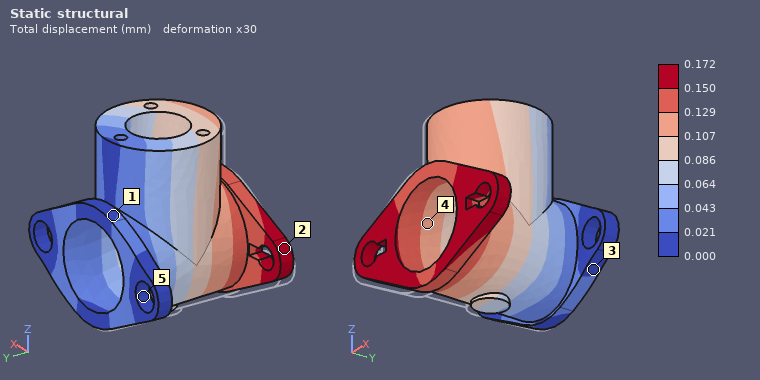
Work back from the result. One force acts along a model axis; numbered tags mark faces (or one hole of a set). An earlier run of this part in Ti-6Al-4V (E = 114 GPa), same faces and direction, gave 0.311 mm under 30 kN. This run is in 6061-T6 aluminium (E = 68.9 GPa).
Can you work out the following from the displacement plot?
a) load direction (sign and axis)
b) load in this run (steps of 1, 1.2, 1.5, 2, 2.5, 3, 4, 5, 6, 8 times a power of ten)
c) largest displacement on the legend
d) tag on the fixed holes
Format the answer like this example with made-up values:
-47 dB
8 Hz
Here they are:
+X
10 kN
0.172 mm
5
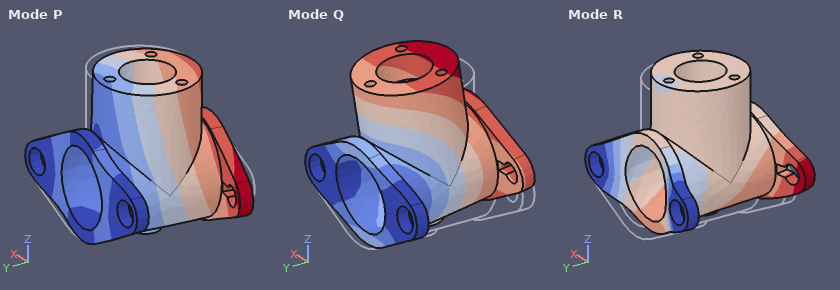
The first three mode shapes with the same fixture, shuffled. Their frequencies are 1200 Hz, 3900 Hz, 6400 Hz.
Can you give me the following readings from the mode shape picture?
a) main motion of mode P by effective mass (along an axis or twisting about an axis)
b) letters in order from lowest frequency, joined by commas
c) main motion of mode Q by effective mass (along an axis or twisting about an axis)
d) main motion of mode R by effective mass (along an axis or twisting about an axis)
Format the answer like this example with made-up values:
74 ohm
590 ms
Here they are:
along X
Q, P, R
along Z
along Y
